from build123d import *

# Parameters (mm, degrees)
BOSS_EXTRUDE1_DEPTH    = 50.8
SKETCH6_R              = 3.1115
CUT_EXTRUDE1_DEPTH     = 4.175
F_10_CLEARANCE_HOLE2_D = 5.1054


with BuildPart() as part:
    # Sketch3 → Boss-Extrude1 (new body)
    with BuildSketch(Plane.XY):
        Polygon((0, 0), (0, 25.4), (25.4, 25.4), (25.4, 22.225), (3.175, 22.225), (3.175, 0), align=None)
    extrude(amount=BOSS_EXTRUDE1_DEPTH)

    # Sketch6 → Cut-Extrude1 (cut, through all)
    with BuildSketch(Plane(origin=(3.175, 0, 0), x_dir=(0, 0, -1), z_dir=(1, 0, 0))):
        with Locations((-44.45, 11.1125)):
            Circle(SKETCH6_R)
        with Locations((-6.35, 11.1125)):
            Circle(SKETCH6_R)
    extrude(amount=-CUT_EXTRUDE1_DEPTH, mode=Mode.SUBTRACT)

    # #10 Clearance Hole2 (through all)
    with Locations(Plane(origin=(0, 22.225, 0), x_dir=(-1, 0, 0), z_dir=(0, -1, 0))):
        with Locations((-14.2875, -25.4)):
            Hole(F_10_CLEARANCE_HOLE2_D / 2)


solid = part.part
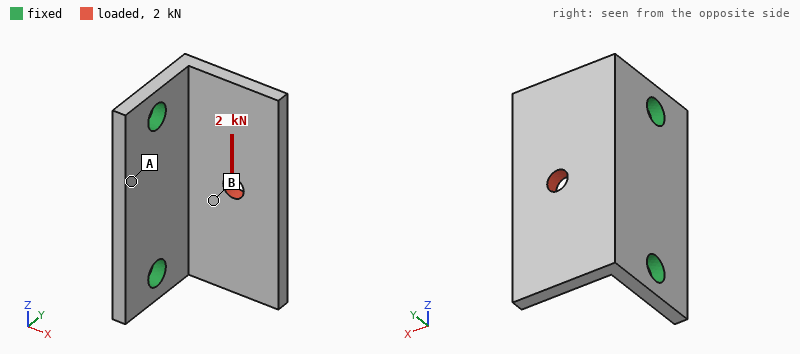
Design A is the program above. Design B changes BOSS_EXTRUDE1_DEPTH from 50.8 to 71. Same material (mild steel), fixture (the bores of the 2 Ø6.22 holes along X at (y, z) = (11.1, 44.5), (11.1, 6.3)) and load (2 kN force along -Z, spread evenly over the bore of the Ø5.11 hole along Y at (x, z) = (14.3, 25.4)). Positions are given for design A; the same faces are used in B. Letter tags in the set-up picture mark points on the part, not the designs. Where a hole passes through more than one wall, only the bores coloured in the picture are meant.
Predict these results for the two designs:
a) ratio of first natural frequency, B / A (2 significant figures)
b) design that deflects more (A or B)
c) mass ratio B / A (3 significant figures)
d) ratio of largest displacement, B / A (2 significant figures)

0.93
B
1.41
1.1
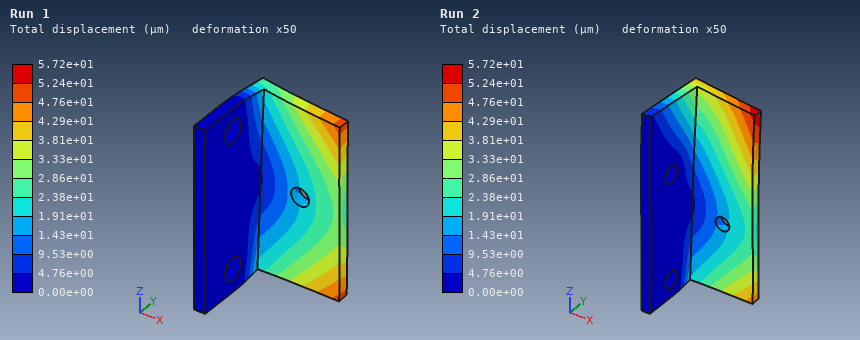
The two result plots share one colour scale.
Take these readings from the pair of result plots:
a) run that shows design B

Run 2
